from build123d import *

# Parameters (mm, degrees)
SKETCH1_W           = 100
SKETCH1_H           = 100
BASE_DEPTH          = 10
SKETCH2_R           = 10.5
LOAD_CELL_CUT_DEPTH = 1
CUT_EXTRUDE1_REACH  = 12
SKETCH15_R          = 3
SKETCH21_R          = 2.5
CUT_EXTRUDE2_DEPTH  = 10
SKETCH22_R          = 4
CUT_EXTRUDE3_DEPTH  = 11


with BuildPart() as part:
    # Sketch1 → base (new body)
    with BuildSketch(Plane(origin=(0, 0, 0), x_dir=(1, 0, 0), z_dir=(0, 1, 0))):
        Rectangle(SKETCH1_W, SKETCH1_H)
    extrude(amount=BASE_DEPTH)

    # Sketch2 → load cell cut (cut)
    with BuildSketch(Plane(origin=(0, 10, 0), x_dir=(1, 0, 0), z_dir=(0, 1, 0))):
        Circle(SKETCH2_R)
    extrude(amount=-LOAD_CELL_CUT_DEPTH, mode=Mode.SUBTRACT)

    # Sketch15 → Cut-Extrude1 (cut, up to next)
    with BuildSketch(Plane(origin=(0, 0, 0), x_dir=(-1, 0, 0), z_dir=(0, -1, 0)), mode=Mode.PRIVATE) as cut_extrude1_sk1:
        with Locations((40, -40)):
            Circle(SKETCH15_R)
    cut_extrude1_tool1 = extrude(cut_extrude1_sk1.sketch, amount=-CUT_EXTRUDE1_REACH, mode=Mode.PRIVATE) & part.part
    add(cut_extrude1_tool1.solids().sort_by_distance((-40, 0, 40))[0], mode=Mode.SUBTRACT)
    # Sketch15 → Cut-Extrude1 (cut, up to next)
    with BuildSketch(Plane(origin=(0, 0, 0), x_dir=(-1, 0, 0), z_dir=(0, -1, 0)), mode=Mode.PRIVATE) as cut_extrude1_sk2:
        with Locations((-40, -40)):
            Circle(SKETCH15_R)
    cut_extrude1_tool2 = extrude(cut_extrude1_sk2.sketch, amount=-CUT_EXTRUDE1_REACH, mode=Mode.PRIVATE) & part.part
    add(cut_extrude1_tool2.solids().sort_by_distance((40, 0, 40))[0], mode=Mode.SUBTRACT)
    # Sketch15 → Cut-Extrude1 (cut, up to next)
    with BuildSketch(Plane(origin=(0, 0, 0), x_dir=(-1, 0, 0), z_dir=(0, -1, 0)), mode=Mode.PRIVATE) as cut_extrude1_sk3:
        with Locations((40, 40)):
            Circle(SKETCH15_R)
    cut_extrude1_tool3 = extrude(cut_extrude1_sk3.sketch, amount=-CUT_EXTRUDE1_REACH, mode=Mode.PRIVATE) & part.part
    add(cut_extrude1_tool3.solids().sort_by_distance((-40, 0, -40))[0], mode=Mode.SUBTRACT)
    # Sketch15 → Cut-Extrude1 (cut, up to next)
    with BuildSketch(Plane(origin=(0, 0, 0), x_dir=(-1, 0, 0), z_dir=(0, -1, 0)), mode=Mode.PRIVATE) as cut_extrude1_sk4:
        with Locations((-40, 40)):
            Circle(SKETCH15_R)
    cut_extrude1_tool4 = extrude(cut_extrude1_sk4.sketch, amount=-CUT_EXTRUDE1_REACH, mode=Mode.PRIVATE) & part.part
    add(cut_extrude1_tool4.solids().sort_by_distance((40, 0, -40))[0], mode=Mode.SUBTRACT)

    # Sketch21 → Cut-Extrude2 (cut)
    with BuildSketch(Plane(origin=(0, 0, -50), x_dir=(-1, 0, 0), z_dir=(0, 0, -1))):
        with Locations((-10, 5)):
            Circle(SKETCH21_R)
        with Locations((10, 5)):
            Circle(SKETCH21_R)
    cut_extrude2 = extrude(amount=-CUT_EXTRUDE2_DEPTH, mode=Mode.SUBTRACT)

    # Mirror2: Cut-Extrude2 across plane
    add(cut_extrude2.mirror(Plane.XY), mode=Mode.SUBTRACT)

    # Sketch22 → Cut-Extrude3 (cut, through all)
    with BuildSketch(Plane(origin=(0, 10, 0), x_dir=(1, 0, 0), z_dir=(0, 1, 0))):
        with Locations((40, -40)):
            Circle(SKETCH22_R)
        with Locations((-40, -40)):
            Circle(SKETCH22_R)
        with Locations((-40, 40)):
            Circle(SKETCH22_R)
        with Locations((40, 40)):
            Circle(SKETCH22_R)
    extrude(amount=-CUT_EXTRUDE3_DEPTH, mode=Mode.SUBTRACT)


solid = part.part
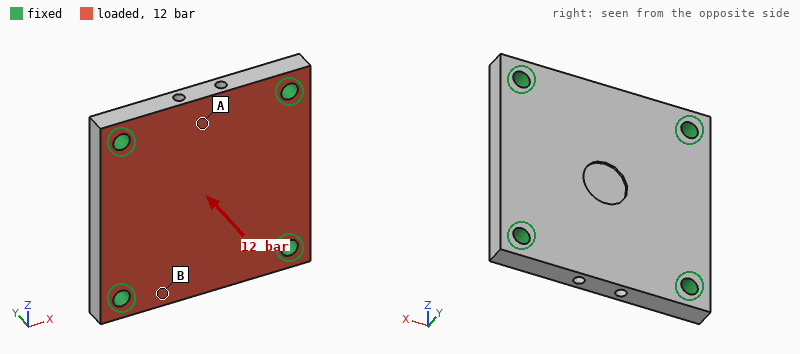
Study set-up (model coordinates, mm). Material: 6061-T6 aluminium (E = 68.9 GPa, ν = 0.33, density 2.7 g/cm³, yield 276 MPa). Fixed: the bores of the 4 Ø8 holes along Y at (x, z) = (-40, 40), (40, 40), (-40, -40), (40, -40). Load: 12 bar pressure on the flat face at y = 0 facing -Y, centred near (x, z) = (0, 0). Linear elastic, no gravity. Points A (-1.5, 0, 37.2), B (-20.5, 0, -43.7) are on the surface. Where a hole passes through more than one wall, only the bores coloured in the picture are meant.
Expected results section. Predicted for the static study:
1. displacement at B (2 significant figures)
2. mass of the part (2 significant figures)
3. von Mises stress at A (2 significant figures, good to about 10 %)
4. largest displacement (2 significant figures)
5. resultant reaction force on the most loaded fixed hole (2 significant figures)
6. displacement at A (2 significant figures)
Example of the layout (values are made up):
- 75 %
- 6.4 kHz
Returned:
- 17 µm
- 260 g
- 23 MPa
- 61 µm
- 2.9 kN
- 36 µm
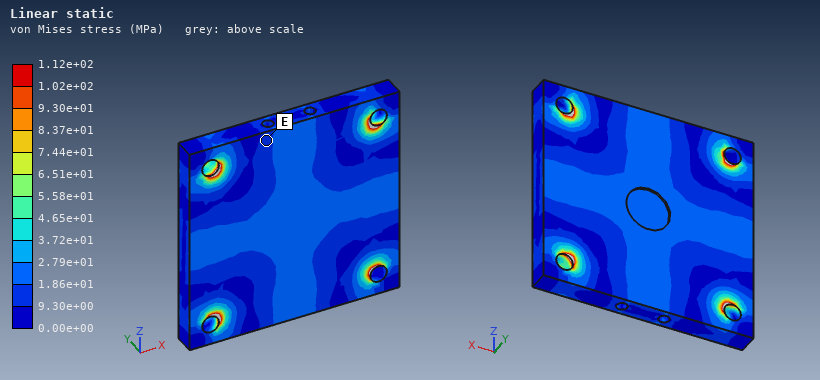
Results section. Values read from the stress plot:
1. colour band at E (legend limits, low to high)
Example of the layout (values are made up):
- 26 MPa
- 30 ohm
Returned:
- 9.30e+00 to 1.86e+01 MPa
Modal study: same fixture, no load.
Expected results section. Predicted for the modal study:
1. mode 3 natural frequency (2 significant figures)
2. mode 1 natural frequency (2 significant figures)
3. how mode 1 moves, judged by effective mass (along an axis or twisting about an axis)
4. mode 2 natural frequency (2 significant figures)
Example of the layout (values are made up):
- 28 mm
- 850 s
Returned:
- 8600 Hz
- 5300 Hz
- along Y
- 8500 Hz
